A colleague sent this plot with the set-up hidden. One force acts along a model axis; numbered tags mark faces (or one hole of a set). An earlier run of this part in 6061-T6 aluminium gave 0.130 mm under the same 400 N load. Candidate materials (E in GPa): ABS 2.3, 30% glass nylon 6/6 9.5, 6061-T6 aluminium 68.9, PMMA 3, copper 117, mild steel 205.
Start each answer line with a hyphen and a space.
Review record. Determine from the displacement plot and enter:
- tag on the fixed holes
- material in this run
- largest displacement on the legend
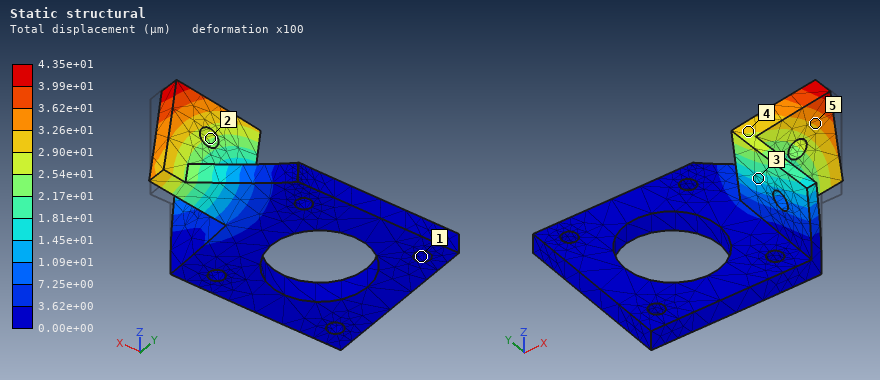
- 1
- mild steel
- 4.35e+01 µm
